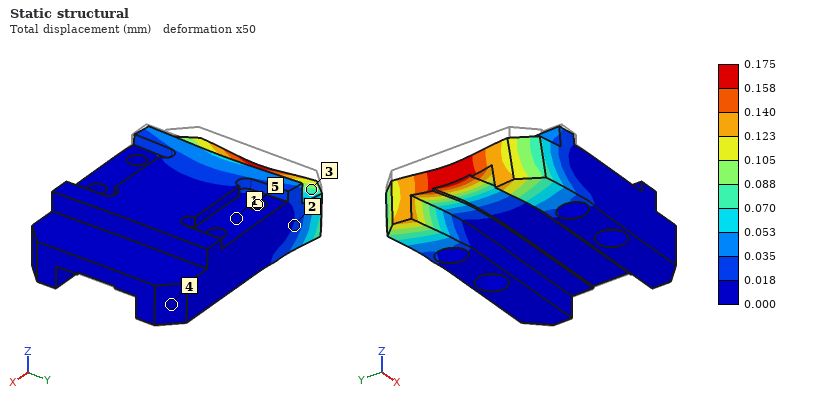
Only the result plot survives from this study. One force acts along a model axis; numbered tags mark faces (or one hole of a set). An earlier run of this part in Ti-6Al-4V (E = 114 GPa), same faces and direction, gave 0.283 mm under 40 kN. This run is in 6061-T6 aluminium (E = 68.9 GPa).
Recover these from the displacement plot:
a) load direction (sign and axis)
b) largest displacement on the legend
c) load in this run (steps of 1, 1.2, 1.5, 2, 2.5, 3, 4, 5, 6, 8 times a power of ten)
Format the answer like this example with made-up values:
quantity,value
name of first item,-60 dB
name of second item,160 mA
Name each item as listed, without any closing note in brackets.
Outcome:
quantity,value
load direction,-Z
largest displacement on the legend,0.175 mm
load in this run,15 kN
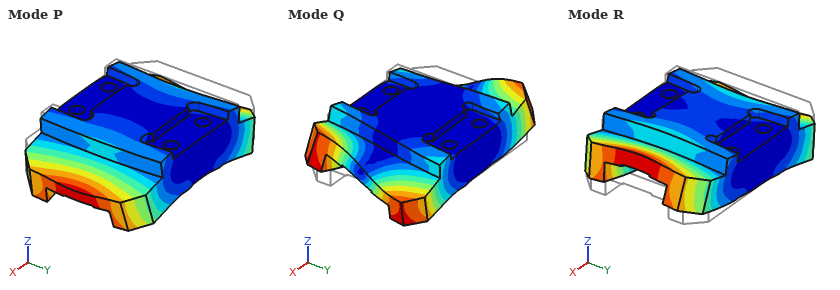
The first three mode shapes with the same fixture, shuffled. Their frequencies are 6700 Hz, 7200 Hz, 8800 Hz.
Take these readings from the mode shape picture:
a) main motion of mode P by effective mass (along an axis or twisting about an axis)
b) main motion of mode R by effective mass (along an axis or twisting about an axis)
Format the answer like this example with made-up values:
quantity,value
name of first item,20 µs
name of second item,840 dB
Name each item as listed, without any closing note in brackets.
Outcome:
quantity,value
main motion of mode P by effective mass,along Z
main motion of mode R by effective mass,twisting about Y
